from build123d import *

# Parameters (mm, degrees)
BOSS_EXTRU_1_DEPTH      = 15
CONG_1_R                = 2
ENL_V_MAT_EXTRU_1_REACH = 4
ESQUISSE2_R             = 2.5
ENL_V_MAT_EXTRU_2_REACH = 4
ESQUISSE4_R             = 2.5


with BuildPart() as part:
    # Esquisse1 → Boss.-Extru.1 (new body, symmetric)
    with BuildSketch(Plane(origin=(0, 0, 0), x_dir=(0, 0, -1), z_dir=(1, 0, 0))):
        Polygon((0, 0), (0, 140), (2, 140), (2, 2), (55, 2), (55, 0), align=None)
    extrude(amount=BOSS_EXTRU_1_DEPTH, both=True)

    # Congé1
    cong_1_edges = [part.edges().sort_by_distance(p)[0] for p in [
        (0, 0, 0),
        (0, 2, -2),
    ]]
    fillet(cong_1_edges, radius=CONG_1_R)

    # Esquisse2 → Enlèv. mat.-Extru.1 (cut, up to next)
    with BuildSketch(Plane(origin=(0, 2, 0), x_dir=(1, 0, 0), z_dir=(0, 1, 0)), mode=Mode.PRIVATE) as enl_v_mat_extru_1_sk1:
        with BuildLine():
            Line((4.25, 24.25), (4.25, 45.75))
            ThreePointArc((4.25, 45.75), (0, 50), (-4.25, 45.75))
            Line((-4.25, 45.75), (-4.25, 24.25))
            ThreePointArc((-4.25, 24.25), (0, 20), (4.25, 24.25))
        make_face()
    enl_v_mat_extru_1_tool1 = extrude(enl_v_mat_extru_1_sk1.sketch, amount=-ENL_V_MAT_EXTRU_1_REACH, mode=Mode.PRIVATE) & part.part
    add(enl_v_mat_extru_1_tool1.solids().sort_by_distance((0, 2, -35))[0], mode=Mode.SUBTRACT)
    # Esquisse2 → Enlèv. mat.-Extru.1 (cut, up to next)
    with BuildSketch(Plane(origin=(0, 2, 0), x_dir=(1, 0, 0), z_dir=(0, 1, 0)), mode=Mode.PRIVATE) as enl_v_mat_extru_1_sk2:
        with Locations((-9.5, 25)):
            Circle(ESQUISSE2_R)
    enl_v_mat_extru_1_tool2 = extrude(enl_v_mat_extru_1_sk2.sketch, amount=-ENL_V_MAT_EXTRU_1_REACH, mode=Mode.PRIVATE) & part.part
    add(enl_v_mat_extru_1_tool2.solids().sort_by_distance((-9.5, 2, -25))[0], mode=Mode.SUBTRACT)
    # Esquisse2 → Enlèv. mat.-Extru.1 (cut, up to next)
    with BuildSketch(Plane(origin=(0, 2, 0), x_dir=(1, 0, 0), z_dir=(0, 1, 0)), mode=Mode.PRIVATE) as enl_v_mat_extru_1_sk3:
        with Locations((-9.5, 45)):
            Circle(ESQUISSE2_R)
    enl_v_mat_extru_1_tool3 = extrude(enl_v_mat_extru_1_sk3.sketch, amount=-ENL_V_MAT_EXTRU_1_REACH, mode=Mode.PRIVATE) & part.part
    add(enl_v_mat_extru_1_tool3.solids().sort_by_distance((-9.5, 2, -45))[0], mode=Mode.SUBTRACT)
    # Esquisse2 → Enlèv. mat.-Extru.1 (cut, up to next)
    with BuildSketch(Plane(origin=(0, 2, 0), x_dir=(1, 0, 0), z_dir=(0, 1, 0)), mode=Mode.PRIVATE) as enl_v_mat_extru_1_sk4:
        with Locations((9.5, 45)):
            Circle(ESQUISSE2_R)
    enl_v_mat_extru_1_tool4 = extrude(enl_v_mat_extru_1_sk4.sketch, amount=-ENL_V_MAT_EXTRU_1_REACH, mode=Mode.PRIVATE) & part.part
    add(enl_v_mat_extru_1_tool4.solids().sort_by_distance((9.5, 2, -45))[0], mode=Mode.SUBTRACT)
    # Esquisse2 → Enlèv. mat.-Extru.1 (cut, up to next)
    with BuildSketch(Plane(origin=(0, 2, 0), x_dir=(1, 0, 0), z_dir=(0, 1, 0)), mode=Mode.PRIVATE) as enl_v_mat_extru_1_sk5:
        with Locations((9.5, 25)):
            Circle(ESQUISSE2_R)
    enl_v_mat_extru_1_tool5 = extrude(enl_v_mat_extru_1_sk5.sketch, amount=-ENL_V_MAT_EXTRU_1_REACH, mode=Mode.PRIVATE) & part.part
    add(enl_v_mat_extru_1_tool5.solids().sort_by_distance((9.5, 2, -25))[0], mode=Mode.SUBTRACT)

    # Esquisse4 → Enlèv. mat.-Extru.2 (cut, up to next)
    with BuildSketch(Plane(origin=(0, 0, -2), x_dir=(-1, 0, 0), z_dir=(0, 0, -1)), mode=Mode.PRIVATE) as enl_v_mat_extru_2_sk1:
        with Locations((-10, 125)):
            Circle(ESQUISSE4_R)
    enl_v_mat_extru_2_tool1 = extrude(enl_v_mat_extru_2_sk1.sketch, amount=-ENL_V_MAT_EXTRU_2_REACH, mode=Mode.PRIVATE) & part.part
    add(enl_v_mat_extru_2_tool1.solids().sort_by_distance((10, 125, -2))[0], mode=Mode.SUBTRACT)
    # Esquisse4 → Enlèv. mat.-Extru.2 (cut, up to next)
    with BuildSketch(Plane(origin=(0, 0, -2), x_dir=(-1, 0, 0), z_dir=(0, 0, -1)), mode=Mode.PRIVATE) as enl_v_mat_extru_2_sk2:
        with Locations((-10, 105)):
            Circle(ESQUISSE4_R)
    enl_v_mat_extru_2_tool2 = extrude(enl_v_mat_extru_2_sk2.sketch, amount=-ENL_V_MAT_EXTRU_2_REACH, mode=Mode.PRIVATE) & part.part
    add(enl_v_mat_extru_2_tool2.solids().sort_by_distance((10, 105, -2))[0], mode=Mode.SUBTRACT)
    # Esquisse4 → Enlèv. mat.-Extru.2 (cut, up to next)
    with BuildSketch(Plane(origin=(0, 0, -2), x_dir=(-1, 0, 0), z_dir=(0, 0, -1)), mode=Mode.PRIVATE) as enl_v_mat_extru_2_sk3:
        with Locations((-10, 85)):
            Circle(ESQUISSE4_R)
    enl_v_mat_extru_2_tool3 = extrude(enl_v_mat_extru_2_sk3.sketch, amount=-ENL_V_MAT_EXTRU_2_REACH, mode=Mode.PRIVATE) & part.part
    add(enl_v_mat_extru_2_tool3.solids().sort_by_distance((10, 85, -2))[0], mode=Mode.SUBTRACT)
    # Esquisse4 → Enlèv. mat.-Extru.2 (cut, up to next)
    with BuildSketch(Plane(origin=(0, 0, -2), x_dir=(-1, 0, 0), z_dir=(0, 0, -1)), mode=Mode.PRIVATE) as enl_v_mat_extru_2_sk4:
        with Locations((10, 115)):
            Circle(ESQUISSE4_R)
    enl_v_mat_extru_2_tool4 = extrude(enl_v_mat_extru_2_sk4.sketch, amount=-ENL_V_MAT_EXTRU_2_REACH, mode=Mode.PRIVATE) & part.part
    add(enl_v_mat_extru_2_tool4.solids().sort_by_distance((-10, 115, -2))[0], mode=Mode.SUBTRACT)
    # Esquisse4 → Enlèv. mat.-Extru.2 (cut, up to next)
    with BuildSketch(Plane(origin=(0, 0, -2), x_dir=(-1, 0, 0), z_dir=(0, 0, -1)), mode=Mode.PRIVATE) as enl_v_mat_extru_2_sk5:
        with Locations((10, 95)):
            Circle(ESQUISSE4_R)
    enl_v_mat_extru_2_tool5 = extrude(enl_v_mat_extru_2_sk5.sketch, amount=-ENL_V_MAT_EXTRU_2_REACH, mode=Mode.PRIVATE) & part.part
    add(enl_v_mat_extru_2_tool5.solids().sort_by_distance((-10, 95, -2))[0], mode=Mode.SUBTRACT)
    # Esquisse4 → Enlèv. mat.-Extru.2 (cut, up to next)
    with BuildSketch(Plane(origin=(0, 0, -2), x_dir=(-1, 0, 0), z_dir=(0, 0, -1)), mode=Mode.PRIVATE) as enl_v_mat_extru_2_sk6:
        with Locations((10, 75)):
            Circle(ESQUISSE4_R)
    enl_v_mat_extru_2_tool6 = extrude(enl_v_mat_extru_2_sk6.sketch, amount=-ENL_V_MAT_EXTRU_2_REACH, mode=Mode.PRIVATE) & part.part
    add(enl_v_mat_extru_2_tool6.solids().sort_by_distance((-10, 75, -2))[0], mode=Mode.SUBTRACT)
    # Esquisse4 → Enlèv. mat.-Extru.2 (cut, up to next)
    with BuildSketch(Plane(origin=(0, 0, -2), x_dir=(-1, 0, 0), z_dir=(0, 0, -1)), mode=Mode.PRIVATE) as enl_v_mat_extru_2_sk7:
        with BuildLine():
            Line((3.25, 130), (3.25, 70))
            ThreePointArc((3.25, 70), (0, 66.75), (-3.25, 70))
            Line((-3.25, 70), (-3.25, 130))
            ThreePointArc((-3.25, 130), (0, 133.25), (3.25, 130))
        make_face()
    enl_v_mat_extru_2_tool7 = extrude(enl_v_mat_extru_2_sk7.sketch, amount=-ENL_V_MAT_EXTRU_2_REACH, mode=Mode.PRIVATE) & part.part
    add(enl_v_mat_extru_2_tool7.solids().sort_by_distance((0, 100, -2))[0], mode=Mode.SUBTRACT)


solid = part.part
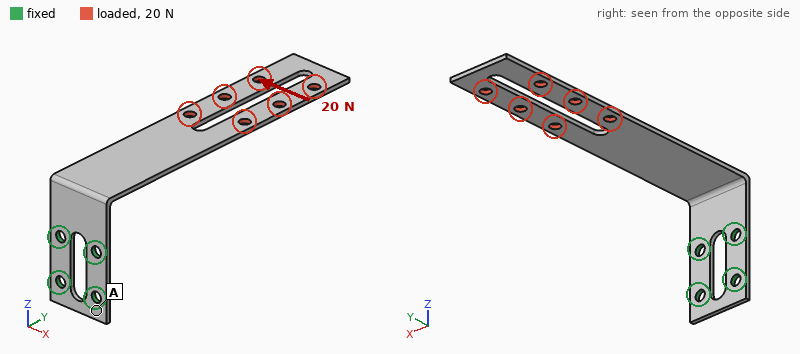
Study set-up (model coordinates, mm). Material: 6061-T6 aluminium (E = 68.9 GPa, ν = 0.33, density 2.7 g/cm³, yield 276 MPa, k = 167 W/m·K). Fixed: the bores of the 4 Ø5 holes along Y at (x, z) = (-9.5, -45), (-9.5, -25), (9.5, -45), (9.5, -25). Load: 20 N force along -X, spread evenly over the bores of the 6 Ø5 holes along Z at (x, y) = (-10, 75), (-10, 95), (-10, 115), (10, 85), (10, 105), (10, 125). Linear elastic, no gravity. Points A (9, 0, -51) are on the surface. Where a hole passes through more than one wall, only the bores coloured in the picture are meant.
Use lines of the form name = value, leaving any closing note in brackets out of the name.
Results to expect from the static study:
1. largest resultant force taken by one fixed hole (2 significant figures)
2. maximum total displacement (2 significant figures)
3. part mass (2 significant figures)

largest resultant force taken by one fixed hole = 87 N
maximum total displacement = 1.6 mm
part mass = 27 g
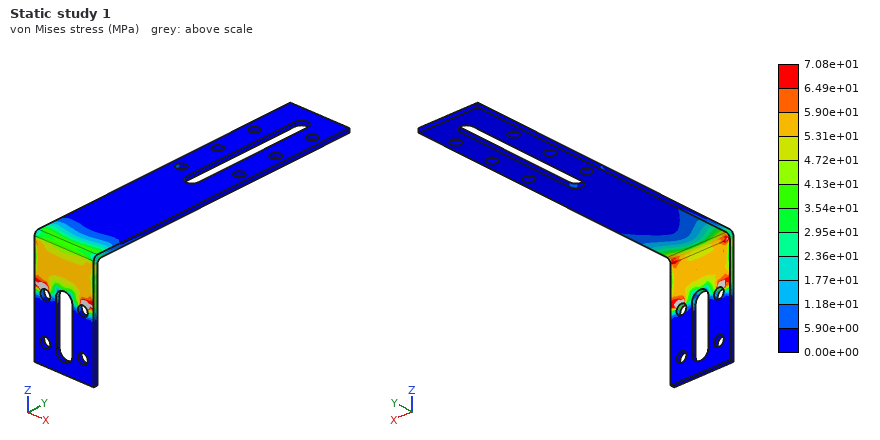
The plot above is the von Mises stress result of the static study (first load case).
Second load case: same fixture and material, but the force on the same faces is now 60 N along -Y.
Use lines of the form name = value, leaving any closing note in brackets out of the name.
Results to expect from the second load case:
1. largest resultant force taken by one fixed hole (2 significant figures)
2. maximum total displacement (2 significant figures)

largest resultant force taken by one fixed hole = 30 N
maximum total displacement = 1.6 mm
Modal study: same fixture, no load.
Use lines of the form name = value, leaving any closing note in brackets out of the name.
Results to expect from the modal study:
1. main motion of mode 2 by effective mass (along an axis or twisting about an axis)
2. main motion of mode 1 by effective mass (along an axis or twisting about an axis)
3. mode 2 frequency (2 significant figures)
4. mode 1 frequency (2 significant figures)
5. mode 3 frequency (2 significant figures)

main motion of mode 2 by effective mass = along X
main motion of mode 1 by effective mass = along Z
mode 2 frequency = 190 Hz
mode 1 frequency = 75 Hz
mode 3 frequency = 420 Hz
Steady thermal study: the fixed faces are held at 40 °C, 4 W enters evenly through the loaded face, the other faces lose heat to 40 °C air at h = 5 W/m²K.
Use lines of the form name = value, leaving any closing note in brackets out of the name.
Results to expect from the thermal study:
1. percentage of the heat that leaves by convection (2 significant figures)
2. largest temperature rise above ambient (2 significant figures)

percentage of the heat that leaves by convection = 28 %
largest temperature rise above ambient = 43 K
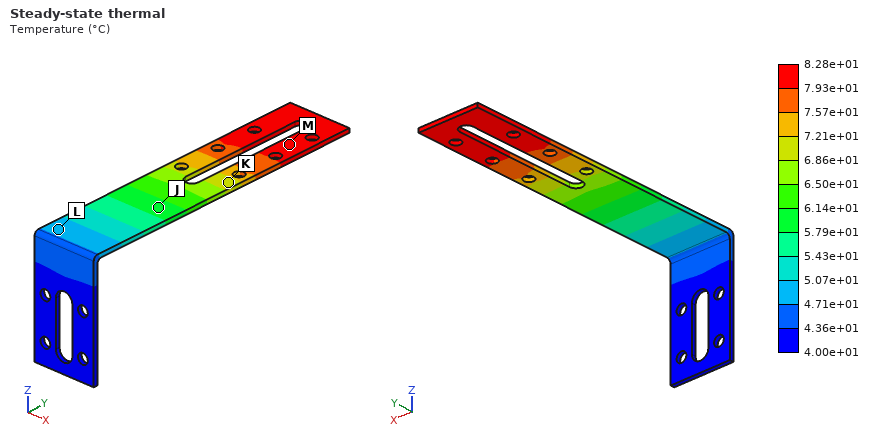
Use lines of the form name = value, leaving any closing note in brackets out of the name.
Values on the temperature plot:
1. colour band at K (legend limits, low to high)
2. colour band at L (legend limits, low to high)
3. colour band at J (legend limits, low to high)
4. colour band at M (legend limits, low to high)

colour band at K = 6.86e+01 to 7.21e+01 °C
colour band at L = 4.71e+01 to 5.07e+01 °C
colour band at J = 5.79e+01 to 6.14e+01 °C
colour band at M = 7.93e+01 to 8.28e+01 °C
